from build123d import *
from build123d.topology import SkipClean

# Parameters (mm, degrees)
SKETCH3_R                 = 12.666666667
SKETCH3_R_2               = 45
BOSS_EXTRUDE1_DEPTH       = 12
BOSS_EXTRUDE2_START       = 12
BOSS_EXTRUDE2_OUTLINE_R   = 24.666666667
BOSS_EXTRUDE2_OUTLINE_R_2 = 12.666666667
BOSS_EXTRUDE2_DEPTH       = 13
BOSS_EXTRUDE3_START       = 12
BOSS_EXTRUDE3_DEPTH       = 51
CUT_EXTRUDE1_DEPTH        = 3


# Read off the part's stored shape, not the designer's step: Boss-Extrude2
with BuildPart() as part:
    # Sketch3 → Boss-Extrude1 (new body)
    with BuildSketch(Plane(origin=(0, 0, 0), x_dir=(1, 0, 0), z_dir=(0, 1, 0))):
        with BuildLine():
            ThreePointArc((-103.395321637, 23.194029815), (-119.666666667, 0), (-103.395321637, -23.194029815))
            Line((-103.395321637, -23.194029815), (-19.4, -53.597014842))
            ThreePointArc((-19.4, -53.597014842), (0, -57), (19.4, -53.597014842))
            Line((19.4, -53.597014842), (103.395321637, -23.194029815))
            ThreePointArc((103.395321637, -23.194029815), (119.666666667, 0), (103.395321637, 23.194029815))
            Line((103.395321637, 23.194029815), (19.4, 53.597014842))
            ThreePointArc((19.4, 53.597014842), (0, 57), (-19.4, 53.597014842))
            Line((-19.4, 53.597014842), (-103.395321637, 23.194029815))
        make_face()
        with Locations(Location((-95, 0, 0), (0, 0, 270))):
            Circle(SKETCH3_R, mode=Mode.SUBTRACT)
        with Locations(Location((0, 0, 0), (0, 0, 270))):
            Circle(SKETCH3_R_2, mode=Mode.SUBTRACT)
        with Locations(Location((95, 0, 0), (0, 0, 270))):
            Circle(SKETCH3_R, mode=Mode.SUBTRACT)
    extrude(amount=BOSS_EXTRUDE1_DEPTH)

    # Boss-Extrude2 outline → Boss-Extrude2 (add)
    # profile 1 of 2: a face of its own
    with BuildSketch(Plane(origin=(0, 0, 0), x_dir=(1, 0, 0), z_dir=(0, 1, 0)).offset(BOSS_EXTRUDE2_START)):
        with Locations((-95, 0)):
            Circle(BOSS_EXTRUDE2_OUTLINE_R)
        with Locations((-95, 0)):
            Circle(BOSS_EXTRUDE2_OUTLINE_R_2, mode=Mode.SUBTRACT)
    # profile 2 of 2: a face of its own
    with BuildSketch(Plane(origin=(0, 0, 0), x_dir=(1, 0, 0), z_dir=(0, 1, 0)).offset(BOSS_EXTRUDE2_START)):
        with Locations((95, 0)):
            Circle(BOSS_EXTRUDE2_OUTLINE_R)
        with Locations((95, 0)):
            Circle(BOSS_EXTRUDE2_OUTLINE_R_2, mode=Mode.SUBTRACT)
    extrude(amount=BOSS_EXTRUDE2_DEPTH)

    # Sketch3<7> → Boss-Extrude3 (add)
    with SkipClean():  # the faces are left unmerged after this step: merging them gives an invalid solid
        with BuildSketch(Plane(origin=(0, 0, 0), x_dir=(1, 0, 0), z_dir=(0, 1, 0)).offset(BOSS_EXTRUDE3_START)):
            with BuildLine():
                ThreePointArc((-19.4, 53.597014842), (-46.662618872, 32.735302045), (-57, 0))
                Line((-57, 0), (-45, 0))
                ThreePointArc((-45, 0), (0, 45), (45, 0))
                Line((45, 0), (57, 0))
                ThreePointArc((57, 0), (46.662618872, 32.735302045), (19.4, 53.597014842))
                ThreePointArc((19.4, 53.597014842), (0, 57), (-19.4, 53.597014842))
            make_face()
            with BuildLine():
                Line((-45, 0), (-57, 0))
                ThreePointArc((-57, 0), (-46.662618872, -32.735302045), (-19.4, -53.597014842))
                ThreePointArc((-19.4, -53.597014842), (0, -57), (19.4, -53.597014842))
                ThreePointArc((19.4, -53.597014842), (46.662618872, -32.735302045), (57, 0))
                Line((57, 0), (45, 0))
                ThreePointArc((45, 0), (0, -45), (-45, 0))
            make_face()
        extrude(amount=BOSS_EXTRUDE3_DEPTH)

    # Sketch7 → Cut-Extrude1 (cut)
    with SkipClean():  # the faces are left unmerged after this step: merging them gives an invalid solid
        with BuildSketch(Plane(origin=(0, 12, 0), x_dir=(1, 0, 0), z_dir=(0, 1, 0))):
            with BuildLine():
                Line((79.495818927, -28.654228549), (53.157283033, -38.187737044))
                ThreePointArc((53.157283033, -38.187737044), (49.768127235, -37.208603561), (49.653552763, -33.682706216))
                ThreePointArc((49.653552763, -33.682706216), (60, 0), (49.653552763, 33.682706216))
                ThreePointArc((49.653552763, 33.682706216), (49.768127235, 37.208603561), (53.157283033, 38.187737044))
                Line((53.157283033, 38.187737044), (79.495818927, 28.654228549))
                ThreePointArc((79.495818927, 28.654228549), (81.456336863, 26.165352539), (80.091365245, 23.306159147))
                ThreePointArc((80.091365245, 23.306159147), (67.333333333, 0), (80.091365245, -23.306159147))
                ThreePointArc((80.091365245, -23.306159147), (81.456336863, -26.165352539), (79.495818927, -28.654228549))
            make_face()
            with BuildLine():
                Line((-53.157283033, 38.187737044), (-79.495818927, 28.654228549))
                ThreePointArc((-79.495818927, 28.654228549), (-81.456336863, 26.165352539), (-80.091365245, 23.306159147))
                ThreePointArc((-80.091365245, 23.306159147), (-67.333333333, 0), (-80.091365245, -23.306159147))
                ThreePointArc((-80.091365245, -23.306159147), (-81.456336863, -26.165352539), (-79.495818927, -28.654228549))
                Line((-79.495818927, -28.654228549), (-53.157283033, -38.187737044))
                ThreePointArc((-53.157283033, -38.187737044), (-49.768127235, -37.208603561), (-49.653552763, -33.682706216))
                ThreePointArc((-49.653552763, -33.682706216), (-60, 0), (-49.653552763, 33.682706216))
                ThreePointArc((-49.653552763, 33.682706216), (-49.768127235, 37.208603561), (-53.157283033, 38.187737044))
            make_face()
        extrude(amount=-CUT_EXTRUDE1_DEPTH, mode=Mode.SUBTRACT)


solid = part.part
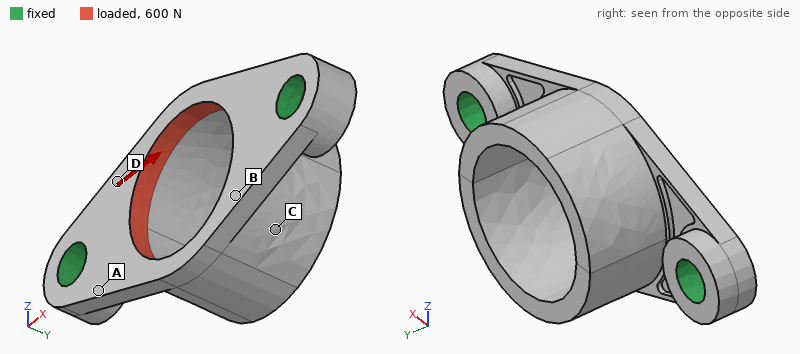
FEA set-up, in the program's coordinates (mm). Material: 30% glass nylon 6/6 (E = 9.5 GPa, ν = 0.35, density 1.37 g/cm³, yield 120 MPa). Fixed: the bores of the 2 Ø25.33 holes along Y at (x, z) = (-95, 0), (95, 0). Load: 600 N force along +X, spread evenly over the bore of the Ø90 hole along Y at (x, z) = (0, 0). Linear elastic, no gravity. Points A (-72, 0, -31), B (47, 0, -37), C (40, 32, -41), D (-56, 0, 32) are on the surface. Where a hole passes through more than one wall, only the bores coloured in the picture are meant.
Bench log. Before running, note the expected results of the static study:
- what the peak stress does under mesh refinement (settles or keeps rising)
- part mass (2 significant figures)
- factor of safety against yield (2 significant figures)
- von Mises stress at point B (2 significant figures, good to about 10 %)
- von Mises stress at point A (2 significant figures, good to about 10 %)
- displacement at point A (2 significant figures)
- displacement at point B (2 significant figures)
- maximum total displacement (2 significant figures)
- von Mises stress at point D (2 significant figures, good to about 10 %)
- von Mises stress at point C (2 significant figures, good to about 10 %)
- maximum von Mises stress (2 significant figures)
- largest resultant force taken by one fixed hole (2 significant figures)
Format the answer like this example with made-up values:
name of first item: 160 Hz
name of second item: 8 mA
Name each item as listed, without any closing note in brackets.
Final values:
what the peak stress does under mesh refinement: settles
part mass: 490 g
factor of safety against yield: 120
von Mises stress at point B: 0.57 MPa
von Mises stress at point A: 0.38 MPa
displacement at point A: 1.9 µm
displacement at point B: 3.4 µm
maximum total displacement: 5.7 µm
von Mises stress at point D: 0.49 MPa
von Mises stress at point C: 0.14 MPa
maximum von Mises stress: 0.97 MPa
largest resultant force taken by one fixed hole: 300 N
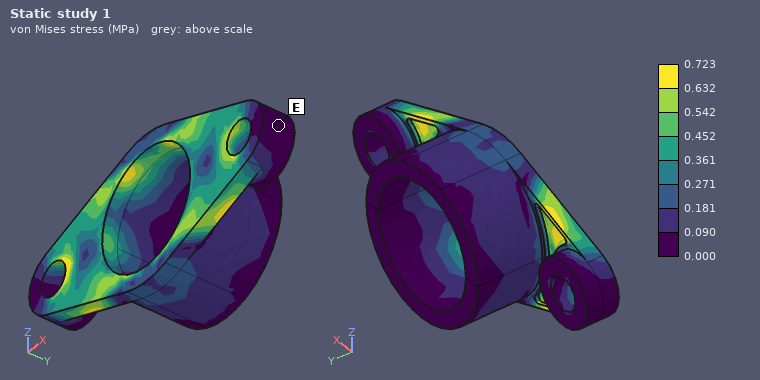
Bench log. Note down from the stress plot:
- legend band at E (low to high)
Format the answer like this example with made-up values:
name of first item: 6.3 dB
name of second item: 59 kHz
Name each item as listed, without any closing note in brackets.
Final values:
legend band at E: 0.000 to 0.090 MPa
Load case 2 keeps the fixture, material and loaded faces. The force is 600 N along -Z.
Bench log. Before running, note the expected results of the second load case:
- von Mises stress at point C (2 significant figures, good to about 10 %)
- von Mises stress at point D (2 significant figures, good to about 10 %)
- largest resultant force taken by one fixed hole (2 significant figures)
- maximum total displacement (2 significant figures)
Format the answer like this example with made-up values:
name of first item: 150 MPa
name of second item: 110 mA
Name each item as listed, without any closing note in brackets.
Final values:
von Mises stress at point C: 0.17 MPa
von Mises stress at point D: 0.52 MPa
largest resultant force taken by one fixed hole: 300 N
maximum total displacement: 11 µm
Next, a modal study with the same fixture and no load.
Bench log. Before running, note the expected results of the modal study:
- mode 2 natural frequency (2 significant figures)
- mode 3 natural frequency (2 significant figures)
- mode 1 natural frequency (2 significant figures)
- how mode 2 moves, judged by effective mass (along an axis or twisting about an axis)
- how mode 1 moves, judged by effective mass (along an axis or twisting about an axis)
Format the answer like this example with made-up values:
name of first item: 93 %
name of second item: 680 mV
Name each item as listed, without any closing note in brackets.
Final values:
mode 2 natural frequency: 1200 Hz
mode 3 natural frequency: 1900 Hz
mode 1 natural frequency: 580 Hz
how mode 2 moves, judged by effective mass: along Y
how mode 1 moves, judged by effective mass: along Z
